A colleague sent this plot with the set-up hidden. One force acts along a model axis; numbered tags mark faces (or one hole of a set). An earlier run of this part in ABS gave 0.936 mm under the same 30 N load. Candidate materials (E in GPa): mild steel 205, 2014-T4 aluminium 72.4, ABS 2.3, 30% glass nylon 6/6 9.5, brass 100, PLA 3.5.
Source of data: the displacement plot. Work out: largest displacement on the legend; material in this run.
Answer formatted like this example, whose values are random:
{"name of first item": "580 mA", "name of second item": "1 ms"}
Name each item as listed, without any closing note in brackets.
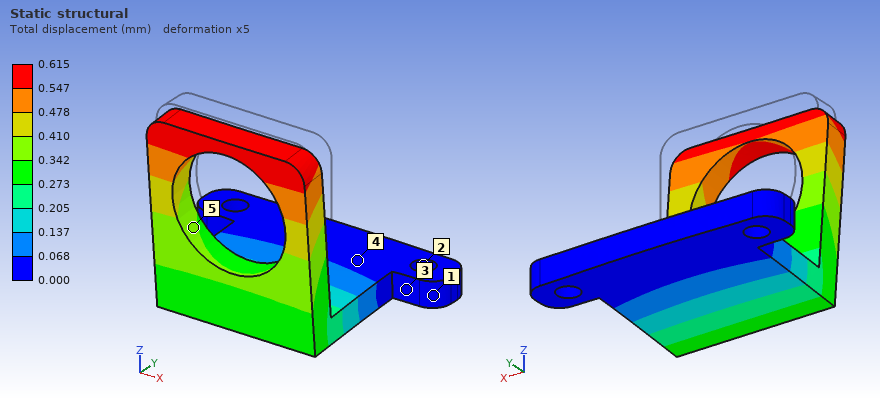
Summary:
{"largest displacement on the legend": "0.615 mm", "material in this run": "PLA"}
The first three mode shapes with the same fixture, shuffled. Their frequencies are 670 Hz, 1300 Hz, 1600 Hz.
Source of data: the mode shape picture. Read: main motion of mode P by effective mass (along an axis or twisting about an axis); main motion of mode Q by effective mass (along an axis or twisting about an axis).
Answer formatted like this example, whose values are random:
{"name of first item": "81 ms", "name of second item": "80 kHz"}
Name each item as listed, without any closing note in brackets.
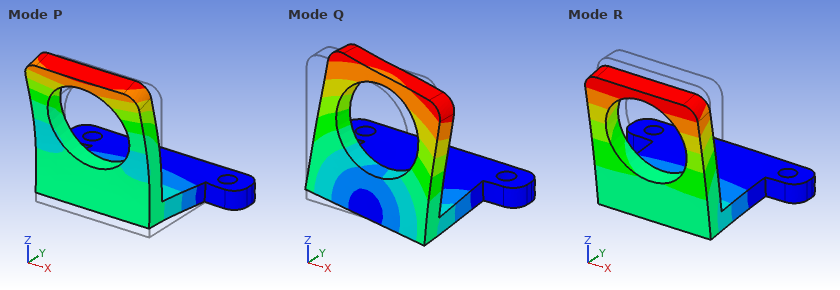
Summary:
{"main motion of mode P by effective mass": "along Z", "main motion of mode Q by effective mass": "along X"}
